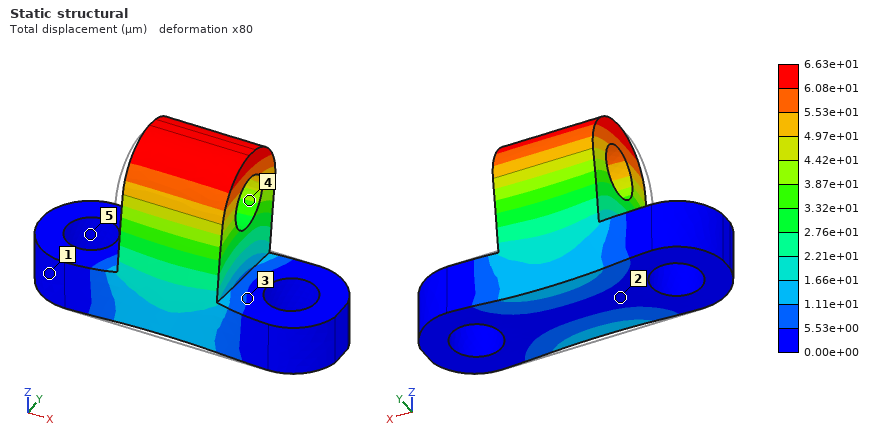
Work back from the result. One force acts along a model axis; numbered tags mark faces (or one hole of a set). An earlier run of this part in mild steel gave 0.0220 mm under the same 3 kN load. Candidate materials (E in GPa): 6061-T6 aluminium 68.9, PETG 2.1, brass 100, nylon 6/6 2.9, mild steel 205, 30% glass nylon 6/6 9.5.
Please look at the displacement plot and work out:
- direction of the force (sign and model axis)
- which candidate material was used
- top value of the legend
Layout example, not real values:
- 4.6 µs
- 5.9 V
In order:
- +Y
- 6061-T6 aluminium
- 6.63e+01 µm
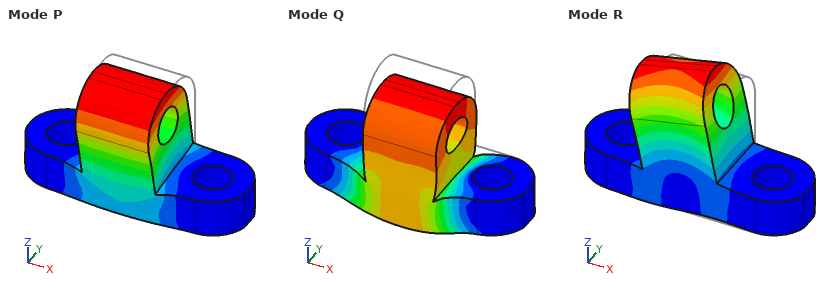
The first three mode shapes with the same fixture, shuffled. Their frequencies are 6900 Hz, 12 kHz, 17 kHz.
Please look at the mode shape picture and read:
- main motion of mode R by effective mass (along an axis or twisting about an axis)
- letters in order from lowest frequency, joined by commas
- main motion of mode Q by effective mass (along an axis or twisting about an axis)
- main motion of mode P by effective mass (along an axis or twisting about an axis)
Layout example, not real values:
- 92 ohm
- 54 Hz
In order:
- along X
- P, R, Q
- along Z
- along Y
